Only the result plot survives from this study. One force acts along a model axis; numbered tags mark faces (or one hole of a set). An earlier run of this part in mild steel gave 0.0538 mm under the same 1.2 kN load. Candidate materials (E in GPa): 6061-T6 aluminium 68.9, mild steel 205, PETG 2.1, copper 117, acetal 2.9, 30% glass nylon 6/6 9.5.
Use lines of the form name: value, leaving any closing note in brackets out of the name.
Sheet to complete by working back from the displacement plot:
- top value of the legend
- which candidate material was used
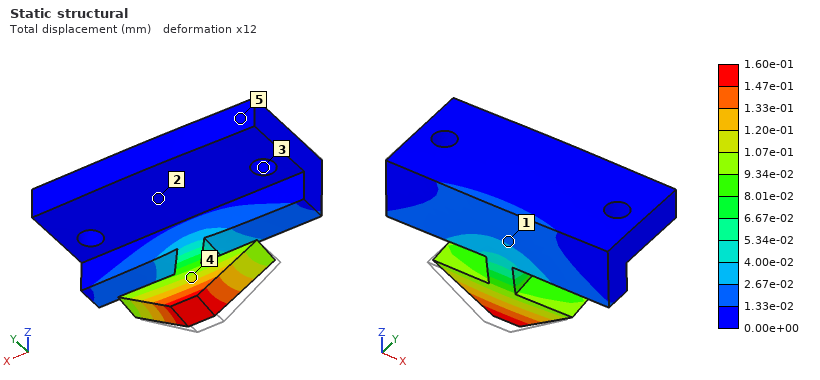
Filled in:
top value of the legend: 1.60e-01 mm
which candidate material was used: 6061-T6 aluminium
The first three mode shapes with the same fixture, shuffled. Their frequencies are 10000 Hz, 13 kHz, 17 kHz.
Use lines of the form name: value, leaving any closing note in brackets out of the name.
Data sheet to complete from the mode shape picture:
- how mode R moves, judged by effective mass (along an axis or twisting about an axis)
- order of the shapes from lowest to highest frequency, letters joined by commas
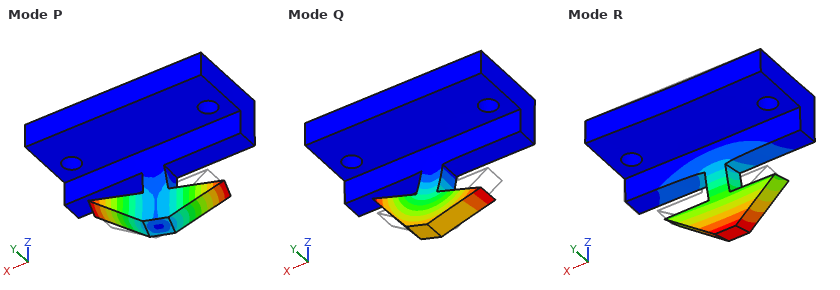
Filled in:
how mode R moves, judged by effective mass: along Y
order of the shapes from lowest to highest frequency, letters joined by commas: R, Q, P
